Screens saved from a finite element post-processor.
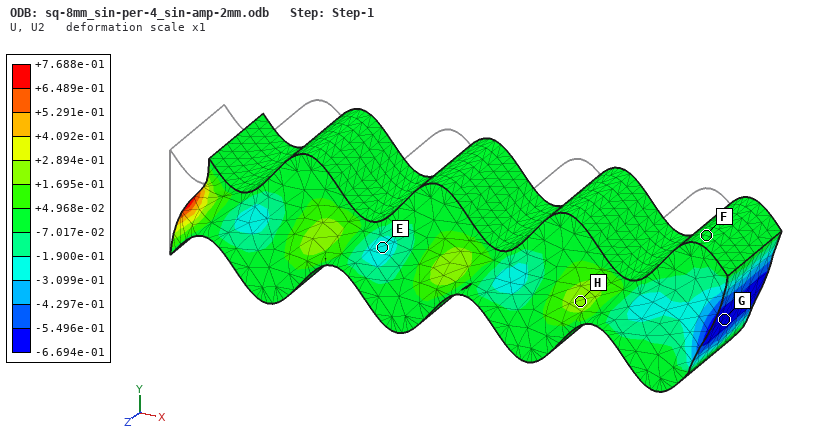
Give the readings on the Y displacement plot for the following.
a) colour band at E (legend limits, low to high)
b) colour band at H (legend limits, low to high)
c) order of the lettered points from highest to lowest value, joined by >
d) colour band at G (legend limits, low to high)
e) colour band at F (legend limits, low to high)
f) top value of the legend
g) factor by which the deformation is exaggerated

-3.099e-01 to -1.900e-01
+1.695e-01 to +2.894e-01
H > F > E > G
-6.694e-01 to -5.496e-01
-7.017e-02 to +4.968e-02
+7.688e-01
1
